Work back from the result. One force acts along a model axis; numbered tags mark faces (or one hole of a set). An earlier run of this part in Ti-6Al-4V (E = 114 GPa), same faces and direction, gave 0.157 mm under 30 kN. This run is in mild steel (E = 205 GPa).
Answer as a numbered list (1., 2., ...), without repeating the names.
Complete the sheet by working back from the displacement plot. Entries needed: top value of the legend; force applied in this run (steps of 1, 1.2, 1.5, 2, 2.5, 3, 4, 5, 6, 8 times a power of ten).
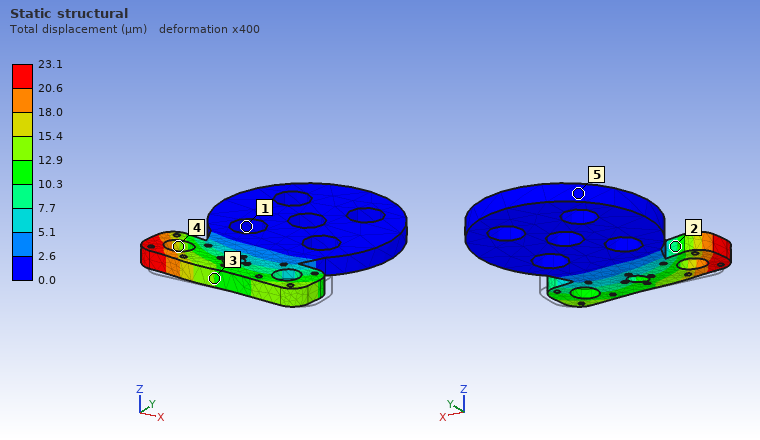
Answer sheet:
1. 23.1 µm
2. 8 kN
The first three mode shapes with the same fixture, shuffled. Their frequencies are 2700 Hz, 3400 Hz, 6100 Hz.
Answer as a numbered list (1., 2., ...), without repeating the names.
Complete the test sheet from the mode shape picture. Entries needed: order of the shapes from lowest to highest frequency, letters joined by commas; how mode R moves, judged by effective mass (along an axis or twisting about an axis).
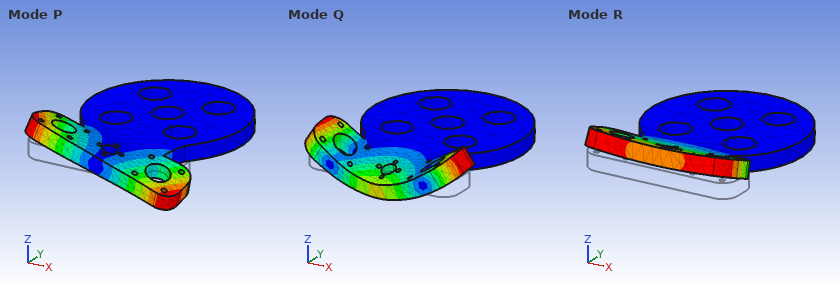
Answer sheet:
1. R, P, Q
2. along Z
